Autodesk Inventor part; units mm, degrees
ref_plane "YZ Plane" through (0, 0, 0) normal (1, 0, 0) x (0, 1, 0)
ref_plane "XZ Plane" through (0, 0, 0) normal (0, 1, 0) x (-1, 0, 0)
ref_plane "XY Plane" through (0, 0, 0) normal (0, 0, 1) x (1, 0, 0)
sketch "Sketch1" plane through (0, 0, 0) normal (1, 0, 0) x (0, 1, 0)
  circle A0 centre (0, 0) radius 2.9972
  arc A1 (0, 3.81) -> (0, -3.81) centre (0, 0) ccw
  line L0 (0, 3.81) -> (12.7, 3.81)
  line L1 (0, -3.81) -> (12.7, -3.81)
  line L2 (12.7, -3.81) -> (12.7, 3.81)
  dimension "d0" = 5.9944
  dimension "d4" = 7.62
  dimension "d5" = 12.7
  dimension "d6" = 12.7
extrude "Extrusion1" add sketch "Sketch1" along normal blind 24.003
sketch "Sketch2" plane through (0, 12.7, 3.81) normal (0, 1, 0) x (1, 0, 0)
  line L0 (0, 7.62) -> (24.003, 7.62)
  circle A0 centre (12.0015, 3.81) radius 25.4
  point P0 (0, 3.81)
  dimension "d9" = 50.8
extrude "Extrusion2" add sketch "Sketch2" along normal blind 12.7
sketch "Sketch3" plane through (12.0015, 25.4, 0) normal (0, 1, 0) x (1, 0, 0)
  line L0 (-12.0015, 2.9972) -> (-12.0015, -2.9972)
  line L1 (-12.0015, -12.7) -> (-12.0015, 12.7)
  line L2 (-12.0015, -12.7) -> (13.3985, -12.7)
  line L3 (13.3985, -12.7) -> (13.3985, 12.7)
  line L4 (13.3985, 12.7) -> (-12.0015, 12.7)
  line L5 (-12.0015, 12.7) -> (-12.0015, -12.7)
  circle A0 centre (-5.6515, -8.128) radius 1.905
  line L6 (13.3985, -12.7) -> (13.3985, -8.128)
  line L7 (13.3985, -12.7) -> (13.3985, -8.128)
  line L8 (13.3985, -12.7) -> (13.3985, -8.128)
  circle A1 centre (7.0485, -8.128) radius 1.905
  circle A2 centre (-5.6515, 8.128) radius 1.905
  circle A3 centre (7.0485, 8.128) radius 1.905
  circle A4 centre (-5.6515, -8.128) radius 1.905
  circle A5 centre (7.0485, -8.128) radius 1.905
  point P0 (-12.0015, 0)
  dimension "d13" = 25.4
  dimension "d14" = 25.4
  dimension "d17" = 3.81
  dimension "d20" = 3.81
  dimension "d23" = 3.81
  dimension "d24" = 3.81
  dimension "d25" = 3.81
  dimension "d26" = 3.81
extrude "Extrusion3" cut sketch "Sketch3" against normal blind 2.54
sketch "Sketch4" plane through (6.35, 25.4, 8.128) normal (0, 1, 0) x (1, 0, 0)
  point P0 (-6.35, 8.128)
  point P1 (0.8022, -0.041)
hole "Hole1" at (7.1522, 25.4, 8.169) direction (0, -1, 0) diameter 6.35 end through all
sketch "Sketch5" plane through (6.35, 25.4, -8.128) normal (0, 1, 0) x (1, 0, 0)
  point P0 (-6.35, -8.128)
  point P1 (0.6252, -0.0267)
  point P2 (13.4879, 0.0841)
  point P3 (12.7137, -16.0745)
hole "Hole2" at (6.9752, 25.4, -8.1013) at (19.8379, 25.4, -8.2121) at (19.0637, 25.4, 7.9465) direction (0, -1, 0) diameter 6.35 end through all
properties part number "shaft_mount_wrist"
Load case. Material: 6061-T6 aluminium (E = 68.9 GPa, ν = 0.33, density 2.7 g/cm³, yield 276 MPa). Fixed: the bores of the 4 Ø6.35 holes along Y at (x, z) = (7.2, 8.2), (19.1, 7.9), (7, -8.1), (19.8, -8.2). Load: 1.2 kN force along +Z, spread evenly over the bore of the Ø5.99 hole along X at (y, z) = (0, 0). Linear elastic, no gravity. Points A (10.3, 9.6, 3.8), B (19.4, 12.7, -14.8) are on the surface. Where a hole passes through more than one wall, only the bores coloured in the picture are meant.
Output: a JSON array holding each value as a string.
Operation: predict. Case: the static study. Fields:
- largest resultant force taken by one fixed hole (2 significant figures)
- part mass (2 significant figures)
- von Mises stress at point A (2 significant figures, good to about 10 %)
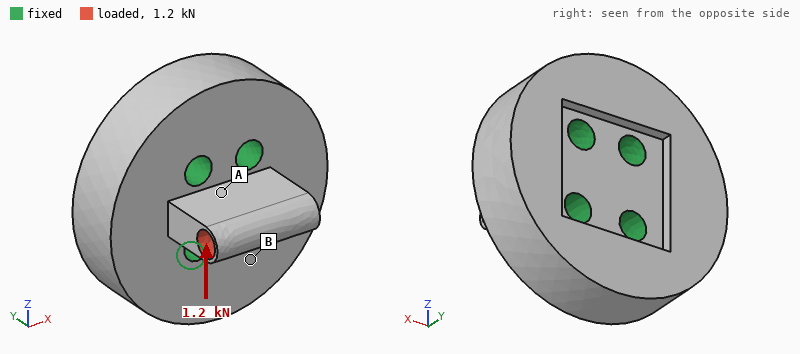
["870 N", "68 g", "45 MPa"]
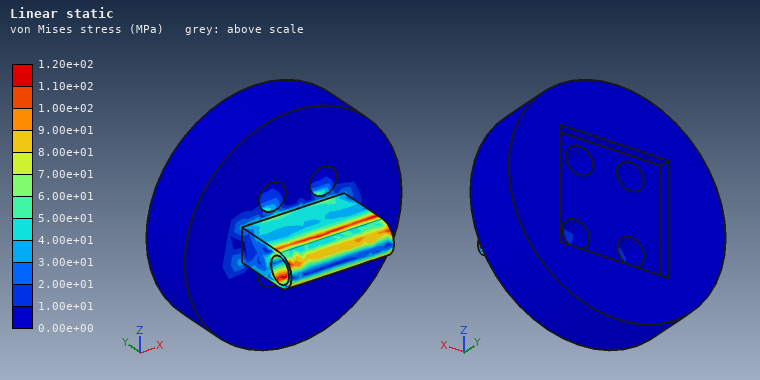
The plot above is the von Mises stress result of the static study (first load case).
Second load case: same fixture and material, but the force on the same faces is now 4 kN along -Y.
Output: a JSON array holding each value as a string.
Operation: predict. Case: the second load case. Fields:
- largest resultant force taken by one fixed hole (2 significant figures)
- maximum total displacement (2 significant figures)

["1.2 kN", "24 µm"]
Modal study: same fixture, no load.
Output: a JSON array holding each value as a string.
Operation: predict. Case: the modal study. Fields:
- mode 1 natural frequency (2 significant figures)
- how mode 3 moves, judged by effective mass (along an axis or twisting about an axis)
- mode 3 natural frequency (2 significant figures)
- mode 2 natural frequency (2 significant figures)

["22 kHz", "twisting about X", "26 kHz", "22 kHz"]
